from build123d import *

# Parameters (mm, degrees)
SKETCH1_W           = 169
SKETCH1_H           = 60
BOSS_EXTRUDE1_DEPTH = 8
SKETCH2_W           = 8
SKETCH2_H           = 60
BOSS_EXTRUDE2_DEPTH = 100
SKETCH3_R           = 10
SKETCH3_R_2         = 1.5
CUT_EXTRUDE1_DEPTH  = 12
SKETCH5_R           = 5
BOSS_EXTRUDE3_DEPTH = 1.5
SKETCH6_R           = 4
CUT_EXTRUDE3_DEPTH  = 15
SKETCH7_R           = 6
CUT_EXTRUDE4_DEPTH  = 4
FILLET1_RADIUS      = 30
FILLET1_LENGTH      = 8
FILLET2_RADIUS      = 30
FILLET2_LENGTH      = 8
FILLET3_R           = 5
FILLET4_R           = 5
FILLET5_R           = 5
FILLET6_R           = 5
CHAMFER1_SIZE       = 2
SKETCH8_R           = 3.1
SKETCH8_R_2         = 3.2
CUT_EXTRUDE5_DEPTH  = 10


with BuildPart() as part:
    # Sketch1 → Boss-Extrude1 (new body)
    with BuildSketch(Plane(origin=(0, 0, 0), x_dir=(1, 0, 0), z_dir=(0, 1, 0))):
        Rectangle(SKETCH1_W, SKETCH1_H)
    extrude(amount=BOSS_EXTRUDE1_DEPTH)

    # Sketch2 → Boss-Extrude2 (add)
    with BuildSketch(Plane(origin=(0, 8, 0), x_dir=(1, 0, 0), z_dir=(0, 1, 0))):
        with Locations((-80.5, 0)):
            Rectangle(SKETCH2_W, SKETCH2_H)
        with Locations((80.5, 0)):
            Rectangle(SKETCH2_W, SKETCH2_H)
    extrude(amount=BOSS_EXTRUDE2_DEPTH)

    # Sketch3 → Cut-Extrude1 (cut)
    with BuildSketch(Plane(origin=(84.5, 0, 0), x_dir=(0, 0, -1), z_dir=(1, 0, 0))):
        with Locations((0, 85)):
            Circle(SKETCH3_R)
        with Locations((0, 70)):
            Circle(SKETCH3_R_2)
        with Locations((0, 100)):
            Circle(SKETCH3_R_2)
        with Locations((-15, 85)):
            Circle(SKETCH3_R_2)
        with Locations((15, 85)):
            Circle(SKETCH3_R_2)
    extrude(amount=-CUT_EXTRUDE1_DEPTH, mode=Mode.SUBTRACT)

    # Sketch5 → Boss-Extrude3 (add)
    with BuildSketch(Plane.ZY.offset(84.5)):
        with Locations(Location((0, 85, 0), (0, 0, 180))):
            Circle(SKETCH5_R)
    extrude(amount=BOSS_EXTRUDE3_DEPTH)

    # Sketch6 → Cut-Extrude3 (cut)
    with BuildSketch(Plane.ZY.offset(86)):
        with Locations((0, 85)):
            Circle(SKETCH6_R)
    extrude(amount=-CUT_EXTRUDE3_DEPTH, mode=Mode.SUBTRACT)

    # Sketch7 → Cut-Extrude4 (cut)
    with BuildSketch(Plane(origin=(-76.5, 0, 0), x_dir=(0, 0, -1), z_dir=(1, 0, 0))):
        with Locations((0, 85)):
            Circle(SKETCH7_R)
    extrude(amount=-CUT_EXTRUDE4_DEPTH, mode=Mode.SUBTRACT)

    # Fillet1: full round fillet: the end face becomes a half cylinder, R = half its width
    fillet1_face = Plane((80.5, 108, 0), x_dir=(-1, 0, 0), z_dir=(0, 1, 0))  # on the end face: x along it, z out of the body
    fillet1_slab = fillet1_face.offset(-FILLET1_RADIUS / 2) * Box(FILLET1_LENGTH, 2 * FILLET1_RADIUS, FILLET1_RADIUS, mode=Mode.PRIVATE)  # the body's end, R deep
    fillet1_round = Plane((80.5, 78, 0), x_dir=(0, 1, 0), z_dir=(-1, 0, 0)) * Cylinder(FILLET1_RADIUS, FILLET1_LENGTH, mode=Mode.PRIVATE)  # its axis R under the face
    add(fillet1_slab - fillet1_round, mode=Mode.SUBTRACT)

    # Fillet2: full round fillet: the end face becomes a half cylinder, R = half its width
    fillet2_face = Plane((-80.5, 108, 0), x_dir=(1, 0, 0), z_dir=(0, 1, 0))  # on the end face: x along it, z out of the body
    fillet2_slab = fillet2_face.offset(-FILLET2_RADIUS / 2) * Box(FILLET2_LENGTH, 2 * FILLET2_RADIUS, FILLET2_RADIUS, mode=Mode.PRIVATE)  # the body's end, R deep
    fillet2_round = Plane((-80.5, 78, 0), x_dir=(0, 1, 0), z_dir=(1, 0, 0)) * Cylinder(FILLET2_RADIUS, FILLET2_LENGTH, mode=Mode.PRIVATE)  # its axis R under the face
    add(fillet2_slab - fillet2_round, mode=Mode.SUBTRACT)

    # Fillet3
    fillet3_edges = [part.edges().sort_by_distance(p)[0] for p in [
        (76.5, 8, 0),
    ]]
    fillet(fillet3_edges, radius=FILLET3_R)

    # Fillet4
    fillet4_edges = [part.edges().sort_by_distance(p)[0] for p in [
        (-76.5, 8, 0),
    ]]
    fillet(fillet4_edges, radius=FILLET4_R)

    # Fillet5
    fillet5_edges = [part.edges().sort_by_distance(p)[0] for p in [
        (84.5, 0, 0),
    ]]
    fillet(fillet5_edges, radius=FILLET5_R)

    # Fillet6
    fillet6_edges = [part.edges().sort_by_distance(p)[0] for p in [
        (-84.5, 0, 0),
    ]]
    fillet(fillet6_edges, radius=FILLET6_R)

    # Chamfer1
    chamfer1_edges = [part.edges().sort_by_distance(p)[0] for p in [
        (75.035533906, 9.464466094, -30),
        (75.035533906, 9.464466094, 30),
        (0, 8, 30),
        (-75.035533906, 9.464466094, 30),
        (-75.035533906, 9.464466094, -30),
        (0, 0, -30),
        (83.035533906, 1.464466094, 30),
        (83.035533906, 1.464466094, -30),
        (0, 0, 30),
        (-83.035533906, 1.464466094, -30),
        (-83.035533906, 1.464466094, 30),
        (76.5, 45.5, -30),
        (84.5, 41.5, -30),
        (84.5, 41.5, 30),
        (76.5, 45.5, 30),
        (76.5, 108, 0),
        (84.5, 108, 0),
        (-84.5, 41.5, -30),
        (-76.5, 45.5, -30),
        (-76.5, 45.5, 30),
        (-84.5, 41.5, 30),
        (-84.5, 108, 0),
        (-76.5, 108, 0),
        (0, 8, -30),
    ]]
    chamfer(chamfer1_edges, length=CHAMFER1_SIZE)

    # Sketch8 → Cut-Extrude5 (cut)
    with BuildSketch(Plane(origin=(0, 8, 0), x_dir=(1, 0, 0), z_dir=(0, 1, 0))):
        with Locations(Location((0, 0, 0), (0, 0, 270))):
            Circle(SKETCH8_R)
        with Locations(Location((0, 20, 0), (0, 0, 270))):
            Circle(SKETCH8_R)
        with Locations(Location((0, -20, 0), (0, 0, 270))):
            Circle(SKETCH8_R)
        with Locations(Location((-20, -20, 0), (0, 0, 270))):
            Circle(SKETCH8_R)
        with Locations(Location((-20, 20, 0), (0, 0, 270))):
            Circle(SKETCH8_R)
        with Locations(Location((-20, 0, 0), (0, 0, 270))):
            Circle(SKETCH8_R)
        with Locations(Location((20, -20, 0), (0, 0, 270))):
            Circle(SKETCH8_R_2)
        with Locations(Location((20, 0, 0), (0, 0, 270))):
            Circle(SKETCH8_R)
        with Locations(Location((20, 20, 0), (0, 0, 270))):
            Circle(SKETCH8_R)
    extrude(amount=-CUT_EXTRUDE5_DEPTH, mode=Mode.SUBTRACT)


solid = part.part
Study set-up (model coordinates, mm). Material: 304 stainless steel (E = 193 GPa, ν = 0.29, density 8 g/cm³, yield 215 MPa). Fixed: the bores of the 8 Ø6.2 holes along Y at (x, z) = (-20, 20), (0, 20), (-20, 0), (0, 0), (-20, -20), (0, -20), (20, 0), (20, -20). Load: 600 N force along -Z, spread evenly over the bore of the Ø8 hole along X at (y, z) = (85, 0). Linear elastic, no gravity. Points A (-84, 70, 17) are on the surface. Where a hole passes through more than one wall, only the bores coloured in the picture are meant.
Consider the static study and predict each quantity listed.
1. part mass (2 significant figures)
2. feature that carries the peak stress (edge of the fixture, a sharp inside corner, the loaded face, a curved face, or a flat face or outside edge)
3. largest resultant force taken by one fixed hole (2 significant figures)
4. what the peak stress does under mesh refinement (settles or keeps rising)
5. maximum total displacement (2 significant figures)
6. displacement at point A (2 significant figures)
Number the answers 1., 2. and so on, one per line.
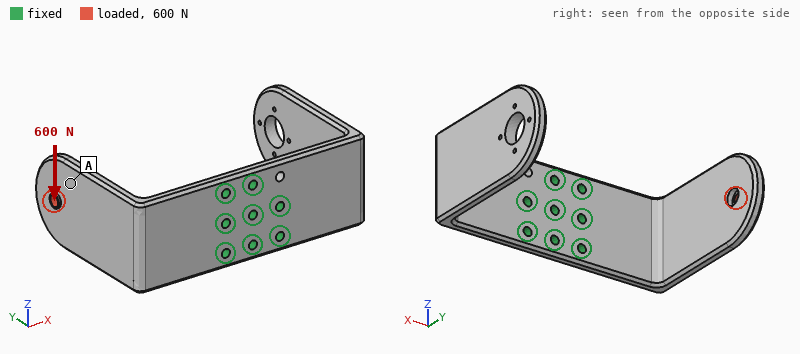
1. 1.3 kg
2. edge of the fixture
3. 1.4 kN
4. keeps rising
5. 0.28 mm
6. 0.18 mm
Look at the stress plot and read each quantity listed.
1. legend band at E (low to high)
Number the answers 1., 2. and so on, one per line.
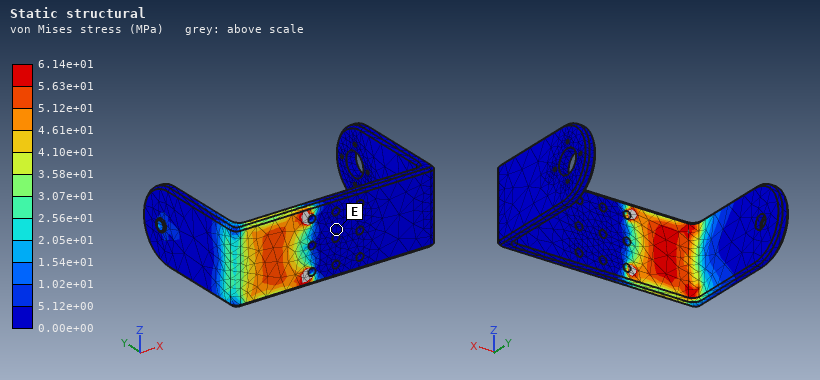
1. 0.00e+00 to 5.12e+00 MPa
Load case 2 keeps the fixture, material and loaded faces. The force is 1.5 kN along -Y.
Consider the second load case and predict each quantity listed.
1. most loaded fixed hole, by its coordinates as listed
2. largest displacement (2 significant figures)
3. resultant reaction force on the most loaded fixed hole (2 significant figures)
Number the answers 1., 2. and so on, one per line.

1. (-20, 0)
2. 0.69 mm
3. 1.2 kN
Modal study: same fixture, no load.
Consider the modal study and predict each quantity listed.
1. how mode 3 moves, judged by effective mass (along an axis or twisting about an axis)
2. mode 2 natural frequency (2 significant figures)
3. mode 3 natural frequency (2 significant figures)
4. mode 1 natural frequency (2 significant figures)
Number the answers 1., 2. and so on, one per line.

1. along Z
2. 350 Hz
3. 580 Hz
4. 340 Hz
